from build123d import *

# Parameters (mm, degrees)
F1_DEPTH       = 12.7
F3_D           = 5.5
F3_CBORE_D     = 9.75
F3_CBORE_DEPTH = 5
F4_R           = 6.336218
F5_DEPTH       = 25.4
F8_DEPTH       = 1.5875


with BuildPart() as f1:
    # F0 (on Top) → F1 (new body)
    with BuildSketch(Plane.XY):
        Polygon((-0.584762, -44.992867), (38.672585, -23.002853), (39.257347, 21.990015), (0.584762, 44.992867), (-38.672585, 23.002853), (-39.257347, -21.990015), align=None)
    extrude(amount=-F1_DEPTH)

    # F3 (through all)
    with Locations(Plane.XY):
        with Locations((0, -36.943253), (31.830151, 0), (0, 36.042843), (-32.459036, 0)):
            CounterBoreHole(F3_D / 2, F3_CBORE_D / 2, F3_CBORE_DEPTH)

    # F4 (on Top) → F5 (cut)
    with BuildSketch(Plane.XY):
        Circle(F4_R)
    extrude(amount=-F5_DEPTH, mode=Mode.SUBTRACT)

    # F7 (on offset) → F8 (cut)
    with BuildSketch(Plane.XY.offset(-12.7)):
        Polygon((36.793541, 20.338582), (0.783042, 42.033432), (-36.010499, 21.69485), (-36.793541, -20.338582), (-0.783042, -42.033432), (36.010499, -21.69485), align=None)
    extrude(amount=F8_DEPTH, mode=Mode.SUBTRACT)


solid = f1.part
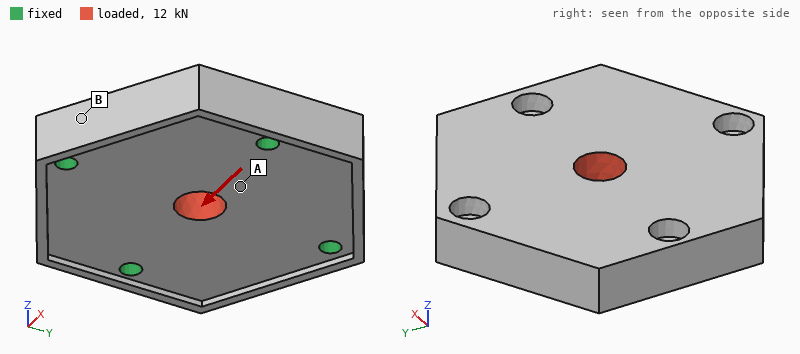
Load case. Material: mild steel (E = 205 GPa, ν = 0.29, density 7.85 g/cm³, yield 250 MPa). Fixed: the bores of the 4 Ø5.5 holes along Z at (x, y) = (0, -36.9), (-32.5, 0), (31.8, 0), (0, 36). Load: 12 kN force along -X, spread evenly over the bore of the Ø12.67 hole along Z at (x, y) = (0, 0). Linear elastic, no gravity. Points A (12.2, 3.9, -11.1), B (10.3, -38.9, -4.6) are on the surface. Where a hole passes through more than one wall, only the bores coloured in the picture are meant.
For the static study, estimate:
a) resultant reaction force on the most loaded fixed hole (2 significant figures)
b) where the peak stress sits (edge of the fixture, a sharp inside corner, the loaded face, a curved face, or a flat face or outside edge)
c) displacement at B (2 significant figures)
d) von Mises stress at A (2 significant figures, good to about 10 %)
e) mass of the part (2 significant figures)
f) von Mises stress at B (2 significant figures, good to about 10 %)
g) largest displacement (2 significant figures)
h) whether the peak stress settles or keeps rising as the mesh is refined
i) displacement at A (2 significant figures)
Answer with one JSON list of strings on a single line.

["4.1 kN", "edge of the fixture", "0.73 µm", "26 MPa", "440 g", "7.6 MPa", "3.8 µm", "keeps rising", "2.7 µm"]
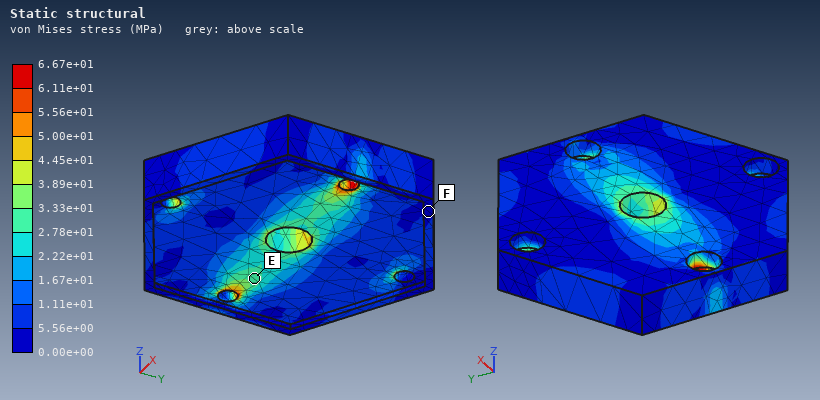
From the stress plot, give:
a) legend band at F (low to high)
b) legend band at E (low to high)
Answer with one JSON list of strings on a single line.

["0.00e+00 to 5.56e+00 MPa", "2.78e+01 to 3.33e+01 MPa"]
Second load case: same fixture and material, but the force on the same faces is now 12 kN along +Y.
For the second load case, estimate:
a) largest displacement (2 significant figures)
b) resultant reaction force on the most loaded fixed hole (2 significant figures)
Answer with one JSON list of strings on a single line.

["3.8 µm", "3.6 kN"]
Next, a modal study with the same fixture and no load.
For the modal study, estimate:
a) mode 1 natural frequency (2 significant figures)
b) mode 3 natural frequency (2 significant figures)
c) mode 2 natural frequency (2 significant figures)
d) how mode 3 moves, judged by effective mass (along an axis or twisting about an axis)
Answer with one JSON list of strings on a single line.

["12 kHz", "13 kHz", "12 kHz", "twisting about X"]
